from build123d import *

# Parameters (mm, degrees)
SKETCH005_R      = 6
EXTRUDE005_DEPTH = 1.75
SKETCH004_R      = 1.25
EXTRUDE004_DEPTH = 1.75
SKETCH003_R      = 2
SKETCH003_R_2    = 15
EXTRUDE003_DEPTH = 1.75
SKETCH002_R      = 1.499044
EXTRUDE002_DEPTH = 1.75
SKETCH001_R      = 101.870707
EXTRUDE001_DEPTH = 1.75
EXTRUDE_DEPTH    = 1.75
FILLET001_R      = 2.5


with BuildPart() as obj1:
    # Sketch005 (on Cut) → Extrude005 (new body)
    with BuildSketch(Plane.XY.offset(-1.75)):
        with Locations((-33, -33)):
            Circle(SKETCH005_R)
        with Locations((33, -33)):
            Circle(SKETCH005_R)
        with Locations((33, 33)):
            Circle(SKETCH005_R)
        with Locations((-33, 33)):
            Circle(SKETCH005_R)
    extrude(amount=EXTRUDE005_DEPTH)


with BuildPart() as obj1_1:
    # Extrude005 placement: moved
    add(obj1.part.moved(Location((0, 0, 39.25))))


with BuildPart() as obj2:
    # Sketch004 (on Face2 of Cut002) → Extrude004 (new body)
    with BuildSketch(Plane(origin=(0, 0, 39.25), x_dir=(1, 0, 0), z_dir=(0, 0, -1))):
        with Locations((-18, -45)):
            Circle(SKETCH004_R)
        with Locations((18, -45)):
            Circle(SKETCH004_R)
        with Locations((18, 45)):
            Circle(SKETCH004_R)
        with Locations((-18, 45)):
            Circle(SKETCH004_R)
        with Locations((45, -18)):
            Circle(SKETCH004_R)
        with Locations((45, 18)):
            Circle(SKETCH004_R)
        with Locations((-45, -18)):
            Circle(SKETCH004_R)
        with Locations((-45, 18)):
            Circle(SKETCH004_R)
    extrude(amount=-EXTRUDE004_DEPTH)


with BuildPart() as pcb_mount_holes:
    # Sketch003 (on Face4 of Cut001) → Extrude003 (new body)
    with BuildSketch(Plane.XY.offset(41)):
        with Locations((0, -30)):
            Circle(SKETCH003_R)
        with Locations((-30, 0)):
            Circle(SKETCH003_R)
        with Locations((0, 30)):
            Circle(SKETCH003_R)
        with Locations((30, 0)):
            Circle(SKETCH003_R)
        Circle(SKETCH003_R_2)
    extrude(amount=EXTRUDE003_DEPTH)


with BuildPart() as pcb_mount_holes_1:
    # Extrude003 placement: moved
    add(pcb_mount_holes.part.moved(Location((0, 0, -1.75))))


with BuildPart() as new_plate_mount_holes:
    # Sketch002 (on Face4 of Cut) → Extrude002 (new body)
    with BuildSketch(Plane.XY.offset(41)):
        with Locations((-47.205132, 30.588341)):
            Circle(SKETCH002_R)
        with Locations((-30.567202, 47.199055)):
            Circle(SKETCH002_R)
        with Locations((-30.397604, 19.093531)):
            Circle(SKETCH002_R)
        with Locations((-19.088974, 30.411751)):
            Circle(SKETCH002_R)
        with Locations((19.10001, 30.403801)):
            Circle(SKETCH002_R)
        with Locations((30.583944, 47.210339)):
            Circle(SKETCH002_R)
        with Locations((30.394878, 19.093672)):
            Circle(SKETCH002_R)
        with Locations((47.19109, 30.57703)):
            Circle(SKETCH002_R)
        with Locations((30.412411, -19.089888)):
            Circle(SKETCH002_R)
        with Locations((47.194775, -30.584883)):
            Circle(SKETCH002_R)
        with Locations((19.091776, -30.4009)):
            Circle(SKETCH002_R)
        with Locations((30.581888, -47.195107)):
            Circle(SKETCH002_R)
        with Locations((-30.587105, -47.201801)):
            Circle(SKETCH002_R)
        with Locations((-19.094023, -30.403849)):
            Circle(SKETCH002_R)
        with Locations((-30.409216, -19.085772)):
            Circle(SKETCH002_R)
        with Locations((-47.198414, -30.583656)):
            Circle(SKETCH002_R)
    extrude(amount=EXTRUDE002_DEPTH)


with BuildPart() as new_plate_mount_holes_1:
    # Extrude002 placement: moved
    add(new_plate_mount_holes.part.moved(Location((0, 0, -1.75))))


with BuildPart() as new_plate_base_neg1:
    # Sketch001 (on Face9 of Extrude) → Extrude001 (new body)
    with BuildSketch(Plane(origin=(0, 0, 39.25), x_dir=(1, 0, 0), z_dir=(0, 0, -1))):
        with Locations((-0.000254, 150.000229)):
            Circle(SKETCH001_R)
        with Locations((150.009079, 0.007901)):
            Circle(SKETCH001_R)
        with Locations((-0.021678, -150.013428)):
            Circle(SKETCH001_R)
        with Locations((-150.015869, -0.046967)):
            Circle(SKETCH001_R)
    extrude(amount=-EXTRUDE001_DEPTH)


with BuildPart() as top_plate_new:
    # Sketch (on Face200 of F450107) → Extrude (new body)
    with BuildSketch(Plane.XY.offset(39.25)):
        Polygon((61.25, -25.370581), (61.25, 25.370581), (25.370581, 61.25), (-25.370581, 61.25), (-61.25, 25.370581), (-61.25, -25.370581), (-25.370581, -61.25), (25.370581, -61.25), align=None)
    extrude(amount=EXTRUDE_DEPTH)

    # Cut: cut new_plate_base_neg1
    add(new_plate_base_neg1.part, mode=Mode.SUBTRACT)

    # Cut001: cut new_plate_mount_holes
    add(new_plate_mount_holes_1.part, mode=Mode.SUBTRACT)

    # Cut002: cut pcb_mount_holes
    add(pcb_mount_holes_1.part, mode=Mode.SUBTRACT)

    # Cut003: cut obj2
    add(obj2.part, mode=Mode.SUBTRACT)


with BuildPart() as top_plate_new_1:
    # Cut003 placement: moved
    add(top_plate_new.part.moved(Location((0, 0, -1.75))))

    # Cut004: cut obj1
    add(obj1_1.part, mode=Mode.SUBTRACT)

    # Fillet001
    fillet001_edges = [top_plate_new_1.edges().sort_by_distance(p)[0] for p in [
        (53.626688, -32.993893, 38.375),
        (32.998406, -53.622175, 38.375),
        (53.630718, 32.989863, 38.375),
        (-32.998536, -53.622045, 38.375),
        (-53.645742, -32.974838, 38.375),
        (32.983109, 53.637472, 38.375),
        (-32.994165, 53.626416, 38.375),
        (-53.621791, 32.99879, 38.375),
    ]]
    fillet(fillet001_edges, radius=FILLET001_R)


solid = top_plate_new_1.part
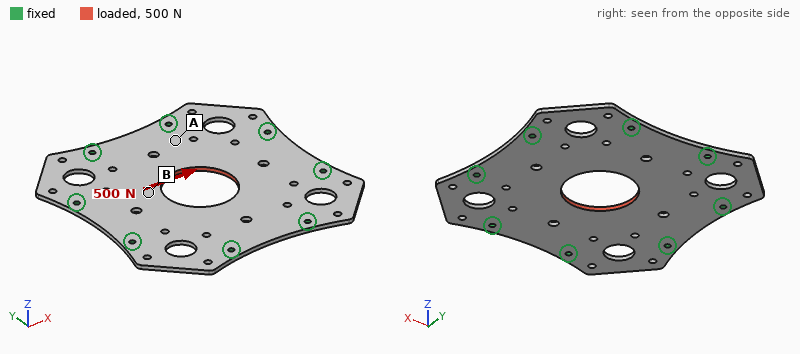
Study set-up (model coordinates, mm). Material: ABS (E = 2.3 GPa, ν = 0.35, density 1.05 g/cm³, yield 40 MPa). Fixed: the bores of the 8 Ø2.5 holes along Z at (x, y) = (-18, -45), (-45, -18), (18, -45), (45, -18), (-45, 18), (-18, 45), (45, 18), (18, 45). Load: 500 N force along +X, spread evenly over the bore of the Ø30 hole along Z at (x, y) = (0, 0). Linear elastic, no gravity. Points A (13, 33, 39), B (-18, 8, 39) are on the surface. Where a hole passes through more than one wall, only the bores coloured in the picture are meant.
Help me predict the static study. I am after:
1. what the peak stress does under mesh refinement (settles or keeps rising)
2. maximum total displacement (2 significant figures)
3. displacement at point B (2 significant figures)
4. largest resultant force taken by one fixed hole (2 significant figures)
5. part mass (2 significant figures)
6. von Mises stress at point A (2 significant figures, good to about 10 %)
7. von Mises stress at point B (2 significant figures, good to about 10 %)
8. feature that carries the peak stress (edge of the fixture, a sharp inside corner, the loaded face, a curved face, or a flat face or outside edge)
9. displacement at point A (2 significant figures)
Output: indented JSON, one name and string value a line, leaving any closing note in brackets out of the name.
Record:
{
  "what the peak stress does under mesh refinement": "keeps rising",
  "maximum total displacement": "54 µm",
  "displacement at point B": "46 µm",
  "largest resultant force taken by one fixed hole": "93 N",
  "part mass": "15 g",
  "von Mises stress at point A": "1.5 MPa",
  "von Mises stress at point B": "3.0 MPa",
  "feature that carries the peak stress": "edge of the fixture",
  "displacement at point A": "16 µm"
}
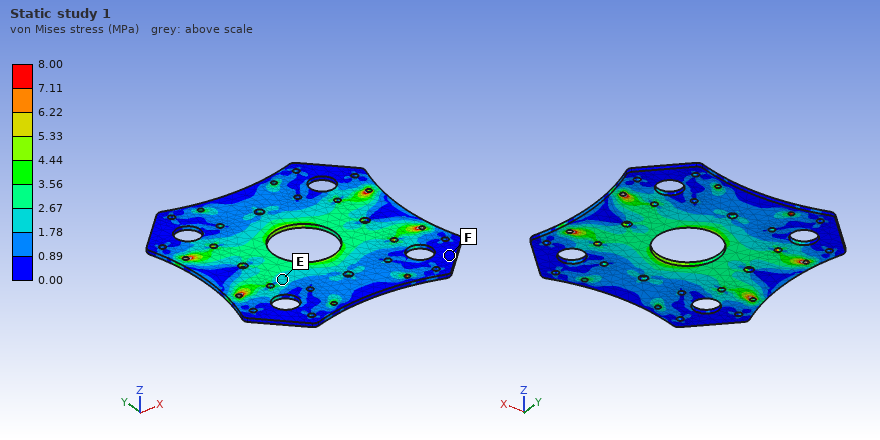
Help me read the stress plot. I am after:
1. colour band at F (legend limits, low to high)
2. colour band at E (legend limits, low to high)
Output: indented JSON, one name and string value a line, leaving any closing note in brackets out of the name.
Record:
{
  "colour band at F": "0.00 to 0.89 MPa",
  "colour band at E": "1.78 to 2.67 MPa"
}
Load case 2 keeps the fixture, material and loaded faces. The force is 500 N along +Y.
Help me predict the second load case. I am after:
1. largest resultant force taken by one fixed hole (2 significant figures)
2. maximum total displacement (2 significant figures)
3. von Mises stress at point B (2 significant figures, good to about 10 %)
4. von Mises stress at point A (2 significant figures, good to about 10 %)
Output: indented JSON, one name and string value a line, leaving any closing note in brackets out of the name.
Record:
{
  "largest resultant force taken by one fixed hole": "93 N",
  "maximum total displacement": "54 µm",
  "von Mises stress at point B": "2.7 MPa",
  "von Mises stress at point A": "3.1 MPa"
}
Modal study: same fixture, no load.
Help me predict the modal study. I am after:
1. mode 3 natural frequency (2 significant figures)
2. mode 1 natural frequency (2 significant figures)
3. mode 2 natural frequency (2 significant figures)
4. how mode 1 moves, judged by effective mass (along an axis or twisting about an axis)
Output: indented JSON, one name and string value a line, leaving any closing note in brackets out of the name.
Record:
{
  "mode 3 natural frequency": "870 Hz",
  "mode 1 natural frequency": "490 Hz",
  "mode 2 natural frequency": "870 Hz",
  "how mode 1 moves, judged by effective mass": "along Z"
}
